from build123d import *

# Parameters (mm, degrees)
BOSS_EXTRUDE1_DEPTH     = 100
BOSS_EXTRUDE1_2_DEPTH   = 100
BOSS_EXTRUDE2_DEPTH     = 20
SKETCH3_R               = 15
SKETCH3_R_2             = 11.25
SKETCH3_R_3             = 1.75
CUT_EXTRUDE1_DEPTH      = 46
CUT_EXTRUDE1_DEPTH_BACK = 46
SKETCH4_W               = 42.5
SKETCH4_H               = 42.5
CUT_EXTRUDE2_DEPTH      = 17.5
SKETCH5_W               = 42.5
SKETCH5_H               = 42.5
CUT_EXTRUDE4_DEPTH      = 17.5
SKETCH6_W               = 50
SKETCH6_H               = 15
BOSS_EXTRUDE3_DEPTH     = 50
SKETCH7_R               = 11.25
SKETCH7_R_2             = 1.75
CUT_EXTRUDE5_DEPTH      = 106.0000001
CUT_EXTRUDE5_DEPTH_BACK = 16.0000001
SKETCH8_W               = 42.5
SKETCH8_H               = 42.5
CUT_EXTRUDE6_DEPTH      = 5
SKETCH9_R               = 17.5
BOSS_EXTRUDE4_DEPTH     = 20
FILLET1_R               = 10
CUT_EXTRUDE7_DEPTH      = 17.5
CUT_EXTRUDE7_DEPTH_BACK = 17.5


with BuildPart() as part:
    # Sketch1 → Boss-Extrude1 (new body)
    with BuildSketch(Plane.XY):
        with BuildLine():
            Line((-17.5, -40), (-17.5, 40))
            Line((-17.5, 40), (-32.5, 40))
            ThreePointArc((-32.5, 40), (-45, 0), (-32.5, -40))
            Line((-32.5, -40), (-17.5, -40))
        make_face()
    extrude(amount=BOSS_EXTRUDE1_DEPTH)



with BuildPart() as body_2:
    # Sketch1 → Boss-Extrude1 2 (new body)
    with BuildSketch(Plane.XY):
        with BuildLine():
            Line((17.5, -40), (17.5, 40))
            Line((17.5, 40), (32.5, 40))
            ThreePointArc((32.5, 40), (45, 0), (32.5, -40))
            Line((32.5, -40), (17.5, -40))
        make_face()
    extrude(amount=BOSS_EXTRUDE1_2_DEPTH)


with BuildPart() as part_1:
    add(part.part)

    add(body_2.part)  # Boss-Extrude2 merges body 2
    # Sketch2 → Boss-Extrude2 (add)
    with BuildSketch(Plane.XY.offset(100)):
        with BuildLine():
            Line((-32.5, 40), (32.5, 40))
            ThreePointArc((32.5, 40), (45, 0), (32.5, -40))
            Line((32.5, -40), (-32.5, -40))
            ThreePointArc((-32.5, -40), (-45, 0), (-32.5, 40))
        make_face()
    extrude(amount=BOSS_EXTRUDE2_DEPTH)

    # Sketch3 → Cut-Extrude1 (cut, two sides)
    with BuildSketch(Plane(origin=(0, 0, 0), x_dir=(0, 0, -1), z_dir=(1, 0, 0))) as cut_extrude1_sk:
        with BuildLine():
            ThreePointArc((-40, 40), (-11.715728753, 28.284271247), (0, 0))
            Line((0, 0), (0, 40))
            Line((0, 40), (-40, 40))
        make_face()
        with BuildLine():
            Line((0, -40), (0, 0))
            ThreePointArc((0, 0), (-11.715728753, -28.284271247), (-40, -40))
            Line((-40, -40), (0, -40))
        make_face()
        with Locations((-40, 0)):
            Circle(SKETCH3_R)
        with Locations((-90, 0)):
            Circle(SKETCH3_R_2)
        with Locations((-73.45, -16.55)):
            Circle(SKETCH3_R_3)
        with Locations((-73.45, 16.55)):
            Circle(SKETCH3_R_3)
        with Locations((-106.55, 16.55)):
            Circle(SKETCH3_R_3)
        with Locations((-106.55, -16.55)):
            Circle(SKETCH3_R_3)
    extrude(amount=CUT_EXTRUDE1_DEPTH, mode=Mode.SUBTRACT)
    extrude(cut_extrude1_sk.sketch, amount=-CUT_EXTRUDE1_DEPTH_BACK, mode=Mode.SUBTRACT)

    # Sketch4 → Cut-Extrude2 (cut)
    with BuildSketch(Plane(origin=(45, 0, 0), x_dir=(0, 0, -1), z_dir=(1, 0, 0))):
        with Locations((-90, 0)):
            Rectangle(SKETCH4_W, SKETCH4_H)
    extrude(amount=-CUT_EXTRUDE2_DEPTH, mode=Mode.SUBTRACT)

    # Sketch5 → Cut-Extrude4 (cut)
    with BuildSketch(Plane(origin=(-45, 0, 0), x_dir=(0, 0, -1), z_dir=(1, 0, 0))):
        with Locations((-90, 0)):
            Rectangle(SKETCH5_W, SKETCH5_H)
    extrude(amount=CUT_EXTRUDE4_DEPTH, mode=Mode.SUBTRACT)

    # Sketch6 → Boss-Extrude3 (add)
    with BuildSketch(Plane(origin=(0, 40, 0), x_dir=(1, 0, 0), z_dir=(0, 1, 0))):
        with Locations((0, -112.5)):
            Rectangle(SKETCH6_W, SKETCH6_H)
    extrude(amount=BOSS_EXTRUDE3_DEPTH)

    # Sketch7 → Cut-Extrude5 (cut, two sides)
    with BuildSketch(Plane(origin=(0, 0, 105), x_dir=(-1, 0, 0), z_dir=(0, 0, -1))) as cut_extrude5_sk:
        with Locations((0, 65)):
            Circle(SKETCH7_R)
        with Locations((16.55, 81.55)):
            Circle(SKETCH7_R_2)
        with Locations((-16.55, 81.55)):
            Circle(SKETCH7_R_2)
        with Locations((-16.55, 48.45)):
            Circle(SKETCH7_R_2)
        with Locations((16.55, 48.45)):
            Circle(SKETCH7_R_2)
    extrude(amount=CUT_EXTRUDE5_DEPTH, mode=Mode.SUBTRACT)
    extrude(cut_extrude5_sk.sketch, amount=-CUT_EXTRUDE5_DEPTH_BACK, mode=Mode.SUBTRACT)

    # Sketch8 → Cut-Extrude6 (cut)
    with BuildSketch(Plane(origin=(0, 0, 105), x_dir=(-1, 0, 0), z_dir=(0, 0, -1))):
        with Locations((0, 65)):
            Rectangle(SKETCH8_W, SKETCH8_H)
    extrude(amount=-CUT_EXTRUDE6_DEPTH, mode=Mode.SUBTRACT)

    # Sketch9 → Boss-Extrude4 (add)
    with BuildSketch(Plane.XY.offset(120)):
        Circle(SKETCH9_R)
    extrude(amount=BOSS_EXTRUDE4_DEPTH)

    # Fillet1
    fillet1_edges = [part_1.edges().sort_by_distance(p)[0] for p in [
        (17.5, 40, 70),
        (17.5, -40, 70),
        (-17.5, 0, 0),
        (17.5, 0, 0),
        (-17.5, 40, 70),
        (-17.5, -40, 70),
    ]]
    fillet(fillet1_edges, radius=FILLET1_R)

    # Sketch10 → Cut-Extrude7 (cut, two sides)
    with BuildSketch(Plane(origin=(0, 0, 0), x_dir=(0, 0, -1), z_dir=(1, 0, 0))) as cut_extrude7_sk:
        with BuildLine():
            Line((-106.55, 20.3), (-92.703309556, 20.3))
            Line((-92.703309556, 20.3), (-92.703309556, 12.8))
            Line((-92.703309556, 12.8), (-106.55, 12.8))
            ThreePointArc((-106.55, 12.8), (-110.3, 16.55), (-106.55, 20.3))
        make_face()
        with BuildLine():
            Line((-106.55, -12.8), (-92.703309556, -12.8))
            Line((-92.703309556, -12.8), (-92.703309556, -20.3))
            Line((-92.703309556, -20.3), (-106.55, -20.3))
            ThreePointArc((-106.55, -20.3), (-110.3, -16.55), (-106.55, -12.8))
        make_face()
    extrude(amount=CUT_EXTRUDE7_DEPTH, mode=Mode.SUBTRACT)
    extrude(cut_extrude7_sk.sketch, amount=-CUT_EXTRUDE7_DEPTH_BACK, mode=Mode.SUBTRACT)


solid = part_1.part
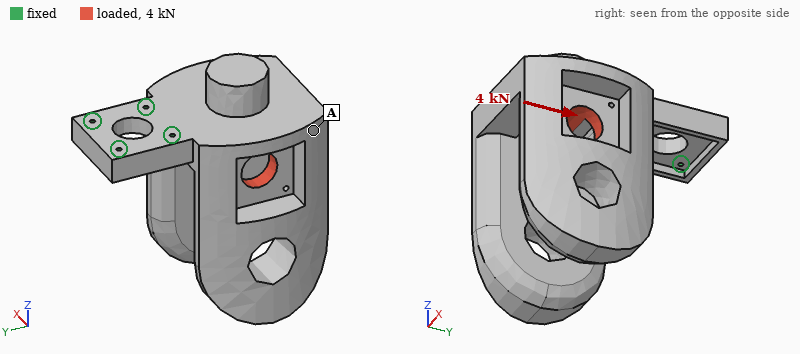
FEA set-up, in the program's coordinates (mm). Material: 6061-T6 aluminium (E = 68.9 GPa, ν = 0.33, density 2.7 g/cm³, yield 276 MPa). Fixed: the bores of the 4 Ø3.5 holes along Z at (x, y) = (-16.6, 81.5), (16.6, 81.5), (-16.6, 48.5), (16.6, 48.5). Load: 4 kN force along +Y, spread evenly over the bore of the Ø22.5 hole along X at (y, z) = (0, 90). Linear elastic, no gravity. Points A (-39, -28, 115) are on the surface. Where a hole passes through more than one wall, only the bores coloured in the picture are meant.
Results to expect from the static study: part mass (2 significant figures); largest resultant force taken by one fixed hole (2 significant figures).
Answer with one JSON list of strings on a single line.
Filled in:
["1.1 kg", "1.6 kN"]
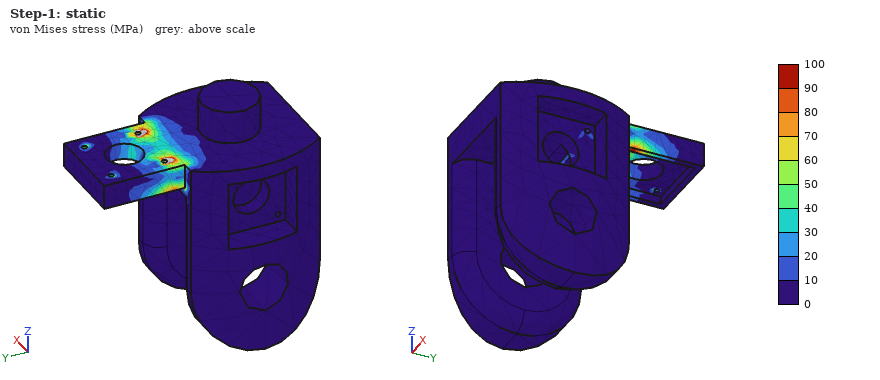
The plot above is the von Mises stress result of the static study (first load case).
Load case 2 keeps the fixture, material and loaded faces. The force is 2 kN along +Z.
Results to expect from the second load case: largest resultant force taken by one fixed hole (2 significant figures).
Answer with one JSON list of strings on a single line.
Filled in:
["1.6 kN"]
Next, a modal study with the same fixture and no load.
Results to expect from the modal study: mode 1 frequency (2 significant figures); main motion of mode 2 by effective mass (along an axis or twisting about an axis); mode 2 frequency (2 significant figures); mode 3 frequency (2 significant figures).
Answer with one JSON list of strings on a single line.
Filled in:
["330 Hz", "along X", "590 Hz", "970 Hz"]
